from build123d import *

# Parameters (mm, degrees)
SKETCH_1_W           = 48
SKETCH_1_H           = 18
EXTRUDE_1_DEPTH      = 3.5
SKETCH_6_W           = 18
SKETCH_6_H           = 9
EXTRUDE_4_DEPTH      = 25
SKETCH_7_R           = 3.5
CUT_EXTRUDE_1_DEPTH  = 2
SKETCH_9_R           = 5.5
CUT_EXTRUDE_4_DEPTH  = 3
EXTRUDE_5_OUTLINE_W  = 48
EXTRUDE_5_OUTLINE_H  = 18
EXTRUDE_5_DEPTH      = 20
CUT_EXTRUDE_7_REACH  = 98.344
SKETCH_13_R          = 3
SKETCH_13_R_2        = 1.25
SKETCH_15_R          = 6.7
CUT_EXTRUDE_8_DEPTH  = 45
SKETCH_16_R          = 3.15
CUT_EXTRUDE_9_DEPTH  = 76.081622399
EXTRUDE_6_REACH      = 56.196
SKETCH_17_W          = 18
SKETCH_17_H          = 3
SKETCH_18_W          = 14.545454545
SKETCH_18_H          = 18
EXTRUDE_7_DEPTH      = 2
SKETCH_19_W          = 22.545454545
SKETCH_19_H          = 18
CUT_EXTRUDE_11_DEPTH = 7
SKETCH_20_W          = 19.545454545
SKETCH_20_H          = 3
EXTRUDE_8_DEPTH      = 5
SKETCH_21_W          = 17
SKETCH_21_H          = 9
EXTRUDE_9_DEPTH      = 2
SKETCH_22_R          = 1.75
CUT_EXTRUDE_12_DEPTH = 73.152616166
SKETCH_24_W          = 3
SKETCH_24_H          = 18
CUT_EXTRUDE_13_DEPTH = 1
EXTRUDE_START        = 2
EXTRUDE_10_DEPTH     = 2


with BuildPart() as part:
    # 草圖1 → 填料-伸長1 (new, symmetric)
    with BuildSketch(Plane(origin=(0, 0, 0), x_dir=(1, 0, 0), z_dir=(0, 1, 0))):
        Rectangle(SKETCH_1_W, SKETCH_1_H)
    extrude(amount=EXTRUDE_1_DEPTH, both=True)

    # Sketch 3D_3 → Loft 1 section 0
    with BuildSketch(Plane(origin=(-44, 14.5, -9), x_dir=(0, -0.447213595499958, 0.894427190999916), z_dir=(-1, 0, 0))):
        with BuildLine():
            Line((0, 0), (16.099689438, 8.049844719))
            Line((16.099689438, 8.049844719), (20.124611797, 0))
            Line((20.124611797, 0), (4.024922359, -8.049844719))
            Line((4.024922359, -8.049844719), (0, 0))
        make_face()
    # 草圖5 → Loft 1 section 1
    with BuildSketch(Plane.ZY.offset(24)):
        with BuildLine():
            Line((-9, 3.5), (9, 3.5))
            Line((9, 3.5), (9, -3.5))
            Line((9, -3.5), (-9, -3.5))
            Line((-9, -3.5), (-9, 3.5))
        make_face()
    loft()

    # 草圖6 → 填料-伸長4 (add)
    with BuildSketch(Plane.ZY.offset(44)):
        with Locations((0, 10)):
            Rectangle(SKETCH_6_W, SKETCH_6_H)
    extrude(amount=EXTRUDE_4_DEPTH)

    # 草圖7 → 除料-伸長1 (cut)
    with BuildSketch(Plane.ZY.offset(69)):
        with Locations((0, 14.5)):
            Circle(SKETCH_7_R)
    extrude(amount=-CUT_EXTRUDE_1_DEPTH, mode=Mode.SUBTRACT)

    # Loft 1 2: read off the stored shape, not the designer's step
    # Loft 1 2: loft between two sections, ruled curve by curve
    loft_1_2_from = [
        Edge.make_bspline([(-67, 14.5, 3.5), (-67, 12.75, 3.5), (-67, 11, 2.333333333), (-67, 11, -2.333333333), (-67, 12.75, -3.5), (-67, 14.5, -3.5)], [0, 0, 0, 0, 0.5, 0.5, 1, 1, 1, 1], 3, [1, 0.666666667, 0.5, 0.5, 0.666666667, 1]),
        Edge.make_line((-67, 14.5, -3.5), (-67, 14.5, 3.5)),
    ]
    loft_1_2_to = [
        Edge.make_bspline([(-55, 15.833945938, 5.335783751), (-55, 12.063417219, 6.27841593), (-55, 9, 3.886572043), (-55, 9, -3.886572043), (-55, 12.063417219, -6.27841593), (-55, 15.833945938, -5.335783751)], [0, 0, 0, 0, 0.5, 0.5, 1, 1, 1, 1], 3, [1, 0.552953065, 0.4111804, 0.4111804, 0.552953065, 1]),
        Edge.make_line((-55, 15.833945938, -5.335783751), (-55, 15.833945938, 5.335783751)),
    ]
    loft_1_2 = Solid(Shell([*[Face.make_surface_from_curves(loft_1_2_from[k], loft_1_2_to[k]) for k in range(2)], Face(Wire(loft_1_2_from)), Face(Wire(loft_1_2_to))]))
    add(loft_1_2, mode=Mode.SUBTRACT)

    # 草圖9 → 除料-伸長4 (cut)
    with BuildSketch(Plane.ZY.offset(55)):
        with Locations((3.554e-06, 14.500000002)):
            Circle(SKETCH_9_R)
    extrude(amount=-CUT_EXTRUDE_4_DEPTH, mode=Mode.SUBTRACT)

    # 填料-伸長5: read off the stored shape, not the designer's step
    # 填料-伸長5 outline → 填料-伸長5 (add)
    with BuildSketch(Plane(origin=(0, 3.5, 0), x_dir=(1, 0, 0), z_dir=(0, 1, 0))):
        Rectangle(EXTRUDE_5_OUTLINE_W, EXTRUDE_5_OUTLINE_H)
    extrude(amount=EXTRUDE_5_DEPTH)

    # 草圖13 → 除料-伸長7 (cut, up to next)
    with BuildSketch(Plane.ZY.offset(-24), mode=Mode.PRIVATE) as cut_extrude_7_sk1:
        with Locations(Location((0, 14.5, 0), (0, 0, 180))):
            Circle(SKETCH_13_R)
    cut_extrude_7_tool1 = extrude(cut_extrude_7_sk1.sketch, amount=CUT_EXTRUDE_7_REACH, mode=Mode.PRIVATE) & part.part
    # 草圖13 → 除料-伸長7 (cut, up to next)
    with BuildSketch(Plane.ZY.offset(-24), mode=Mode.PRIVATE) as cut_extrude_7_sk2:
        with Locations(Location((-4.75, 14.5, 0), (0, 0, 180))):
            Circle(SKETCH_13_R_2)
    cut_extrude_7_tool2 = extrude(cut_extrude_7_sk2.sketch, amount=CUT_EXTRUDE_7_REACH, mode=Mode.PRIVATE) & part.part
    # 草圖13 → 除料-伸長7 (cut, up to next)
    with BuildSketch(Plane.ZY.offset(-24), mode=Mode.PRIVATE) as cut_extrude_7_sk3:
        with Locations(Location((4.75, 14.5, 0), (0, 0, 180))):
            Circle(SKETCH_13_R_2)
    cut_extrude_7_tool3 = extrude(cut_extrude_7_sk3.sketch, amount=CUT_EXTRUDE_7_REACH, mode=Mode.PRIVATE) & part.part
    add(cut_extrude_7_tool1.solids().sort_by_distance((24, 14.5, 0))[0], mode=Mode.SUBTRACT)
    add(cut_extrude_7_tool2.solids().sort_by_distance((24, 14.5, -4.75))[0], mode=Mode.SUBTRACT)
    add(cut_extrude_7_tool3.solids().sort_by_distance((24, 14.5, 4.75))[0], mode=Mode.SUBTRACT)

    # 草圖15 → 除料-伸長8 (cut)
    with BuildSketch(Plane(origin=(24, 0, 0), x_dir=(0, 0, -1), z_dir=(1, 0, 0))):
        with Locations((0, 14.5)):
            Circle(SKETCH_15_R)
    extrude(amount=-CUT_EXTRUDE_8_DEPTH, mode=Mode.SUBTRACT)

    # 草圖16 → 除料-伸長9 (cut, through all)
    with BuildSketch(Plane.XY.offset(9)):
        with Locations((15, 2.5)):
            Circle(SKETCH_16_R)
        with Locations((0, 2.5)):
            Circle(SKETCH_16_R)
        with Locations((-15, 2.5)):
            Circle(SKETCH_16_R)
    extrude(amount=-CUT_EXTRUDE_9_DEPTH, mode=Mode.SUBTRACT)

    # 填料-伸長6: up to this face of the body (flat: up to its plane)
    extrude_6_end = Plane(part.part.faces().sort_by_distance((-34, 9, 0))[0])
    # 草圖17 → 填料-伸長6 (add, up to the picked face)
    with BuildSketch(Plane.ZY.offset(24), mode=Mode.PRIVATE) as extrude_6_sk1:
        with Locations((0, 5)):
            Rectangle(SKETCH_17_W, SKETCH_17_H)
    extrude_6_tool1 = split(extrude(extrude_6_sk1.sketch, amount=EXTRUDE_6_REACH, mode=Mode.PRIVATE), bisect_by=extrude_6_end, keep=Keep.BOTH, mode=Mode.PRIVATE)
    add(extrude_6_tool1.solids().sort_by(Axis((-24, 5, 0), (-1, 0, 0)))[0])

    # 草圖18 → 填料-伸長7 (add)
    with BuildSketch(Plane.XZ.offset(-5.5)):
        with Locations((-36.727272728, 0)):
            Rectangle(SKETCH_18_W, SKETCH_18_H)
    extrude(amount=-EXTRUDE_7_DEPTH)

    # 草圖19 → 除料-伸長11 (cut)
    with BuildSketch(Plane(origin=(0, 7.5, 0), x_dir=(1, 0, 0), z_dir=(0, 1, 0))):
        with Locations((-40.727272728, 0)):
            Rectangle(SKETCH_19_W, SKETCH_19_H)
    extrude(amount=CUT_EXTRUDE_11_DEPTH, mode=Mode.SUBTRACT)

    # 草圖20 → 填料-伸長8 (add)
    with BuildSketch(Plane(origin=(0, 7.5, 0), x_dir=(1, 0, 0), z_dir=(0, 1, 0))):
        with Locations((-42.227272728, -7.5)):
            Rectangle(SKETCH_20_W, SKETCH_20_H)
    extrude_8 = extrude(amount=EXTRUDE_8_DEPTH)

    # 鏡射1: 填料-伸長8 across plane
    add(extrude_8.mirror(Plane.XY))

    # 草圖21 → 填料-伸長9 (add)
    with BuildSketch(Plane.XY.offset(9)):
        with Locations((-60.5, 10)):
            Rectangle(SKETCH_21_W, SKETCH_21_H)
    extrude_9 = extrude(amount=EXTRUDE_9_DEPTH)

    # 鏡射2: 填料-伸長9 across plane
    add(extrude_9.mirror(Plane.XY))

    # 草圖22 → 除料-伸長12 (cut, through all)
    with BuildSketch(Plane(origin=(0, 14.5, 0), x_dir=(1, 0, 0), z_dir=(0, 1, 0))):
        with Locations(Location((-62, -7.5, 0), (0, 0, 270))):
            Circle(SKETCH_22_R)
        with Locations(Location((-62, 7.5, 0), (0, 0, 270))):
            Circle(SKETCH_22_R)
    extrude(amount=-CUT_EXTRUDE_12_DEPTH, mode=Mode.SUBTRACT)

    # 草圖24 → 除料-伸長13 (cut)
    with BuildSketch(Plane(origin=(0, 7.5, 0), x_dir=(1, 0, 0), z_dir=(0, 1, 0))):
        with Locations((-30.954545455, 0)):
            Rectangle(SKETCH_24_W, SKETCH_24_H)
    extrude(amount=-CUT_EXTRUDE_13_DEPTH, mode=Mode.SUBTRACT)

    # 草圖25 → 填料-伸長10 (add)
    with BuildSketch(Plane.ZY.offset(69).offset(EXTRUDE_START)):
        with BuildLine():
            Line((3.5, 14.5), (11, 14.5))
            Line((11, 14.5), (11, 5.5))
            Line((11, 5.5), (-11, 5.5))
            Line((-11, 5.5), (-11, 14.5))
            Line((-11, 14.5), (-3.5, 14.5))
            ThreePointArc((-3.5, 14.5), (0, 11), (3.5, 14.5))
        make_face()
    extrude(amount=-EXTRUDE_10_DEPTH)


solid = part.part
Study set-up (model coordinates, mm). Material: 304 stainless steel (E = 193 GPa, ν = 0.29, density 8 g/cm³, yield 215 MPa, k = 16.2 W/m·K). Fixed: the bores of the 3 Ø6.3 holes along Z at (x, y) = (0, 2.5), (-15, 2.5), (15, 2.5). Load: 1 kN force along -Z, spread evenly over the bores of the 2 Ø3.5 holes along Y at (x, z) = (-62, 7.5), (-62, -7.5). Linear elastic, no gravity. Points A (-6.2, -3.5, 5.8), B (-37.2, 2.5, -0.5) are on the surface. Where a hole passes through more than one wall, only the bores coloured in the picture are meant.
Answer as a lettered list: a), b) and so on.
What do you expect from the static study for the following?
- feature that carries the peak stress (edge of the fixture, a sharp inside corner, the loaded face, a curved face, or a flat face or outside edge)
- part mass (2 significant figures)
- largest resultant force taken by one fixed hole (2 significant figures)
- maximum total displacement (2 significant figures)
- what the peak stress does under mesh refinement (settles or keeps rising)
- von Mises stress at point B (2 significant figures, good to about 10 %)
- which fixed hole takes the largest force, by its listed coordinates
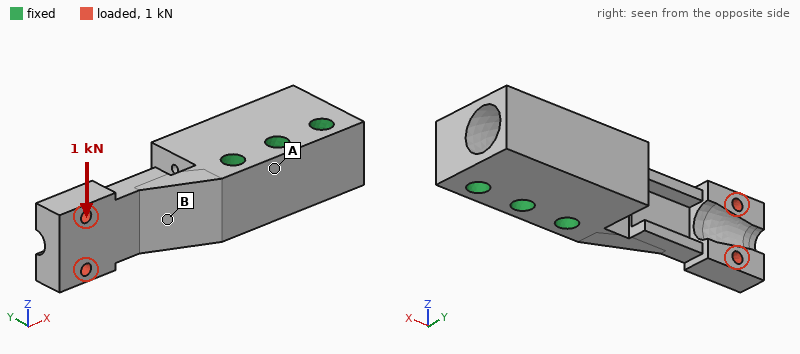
a) a sharp inside corner
b) 170 g
c) 1.1 kN
d) 80 µm
e) keeps rising
f) 61 MPa
g) (-15, 2.5)
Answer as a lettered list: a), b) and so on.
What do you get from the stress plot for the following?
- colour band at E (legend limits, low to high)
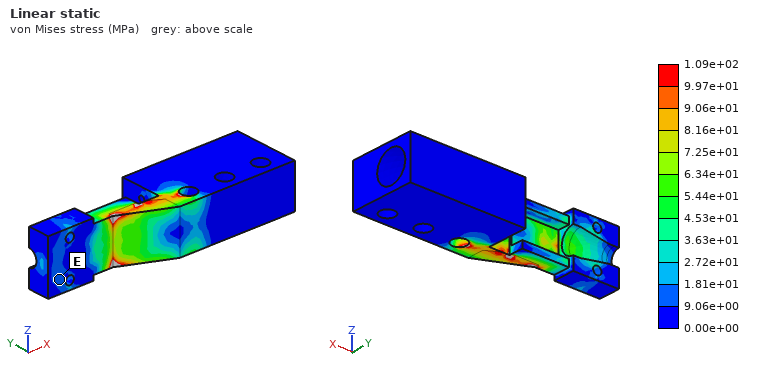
a) 9.06e+00 to 1.81e+01 MPa
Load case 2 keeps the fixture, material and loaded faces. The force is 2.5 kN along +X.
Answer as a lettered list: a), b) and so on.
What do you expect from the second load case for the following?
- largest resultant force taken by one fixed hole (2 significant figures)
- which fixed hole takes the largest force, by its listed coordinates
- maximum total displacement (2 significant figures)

a) 2.2 kN
b) (-15, 2.5)
c) 0.17 mm
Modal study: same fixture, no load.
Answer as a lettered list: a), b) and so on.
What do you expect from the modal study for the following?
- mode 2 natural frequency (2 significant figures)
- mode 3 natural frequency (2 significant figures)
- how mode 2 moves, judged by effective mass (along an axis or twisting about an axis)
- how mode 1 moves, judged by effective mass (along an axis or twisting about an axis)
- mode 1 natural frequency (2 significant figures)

a) 4000 Hz
b) 5200 Hz
c) along Z
d) along Y
e) 1900 Hz
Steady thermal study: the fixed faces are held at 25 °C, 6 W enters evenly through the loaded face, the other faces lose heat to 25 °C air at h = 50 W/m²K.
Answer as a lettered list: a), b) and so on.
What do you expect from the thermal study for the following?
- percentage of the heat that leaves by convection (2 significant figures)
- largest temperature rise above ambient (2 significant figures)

a) 80 %
b) 53 K
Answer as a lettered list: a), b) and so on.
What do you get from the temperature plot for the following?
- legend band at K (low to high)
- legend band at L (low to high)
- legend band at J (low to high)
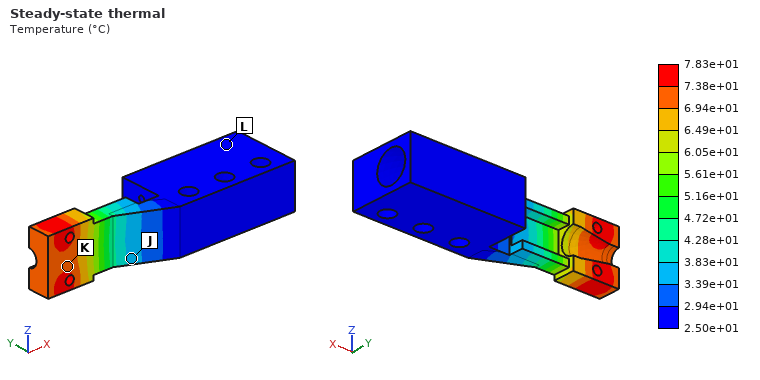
a) 6.94e+01 to 7.38e+01 °C
b) 2.50e+01 to 2.94e+01 °C
c) 3.39e+01 to 3.83e+01 °C
